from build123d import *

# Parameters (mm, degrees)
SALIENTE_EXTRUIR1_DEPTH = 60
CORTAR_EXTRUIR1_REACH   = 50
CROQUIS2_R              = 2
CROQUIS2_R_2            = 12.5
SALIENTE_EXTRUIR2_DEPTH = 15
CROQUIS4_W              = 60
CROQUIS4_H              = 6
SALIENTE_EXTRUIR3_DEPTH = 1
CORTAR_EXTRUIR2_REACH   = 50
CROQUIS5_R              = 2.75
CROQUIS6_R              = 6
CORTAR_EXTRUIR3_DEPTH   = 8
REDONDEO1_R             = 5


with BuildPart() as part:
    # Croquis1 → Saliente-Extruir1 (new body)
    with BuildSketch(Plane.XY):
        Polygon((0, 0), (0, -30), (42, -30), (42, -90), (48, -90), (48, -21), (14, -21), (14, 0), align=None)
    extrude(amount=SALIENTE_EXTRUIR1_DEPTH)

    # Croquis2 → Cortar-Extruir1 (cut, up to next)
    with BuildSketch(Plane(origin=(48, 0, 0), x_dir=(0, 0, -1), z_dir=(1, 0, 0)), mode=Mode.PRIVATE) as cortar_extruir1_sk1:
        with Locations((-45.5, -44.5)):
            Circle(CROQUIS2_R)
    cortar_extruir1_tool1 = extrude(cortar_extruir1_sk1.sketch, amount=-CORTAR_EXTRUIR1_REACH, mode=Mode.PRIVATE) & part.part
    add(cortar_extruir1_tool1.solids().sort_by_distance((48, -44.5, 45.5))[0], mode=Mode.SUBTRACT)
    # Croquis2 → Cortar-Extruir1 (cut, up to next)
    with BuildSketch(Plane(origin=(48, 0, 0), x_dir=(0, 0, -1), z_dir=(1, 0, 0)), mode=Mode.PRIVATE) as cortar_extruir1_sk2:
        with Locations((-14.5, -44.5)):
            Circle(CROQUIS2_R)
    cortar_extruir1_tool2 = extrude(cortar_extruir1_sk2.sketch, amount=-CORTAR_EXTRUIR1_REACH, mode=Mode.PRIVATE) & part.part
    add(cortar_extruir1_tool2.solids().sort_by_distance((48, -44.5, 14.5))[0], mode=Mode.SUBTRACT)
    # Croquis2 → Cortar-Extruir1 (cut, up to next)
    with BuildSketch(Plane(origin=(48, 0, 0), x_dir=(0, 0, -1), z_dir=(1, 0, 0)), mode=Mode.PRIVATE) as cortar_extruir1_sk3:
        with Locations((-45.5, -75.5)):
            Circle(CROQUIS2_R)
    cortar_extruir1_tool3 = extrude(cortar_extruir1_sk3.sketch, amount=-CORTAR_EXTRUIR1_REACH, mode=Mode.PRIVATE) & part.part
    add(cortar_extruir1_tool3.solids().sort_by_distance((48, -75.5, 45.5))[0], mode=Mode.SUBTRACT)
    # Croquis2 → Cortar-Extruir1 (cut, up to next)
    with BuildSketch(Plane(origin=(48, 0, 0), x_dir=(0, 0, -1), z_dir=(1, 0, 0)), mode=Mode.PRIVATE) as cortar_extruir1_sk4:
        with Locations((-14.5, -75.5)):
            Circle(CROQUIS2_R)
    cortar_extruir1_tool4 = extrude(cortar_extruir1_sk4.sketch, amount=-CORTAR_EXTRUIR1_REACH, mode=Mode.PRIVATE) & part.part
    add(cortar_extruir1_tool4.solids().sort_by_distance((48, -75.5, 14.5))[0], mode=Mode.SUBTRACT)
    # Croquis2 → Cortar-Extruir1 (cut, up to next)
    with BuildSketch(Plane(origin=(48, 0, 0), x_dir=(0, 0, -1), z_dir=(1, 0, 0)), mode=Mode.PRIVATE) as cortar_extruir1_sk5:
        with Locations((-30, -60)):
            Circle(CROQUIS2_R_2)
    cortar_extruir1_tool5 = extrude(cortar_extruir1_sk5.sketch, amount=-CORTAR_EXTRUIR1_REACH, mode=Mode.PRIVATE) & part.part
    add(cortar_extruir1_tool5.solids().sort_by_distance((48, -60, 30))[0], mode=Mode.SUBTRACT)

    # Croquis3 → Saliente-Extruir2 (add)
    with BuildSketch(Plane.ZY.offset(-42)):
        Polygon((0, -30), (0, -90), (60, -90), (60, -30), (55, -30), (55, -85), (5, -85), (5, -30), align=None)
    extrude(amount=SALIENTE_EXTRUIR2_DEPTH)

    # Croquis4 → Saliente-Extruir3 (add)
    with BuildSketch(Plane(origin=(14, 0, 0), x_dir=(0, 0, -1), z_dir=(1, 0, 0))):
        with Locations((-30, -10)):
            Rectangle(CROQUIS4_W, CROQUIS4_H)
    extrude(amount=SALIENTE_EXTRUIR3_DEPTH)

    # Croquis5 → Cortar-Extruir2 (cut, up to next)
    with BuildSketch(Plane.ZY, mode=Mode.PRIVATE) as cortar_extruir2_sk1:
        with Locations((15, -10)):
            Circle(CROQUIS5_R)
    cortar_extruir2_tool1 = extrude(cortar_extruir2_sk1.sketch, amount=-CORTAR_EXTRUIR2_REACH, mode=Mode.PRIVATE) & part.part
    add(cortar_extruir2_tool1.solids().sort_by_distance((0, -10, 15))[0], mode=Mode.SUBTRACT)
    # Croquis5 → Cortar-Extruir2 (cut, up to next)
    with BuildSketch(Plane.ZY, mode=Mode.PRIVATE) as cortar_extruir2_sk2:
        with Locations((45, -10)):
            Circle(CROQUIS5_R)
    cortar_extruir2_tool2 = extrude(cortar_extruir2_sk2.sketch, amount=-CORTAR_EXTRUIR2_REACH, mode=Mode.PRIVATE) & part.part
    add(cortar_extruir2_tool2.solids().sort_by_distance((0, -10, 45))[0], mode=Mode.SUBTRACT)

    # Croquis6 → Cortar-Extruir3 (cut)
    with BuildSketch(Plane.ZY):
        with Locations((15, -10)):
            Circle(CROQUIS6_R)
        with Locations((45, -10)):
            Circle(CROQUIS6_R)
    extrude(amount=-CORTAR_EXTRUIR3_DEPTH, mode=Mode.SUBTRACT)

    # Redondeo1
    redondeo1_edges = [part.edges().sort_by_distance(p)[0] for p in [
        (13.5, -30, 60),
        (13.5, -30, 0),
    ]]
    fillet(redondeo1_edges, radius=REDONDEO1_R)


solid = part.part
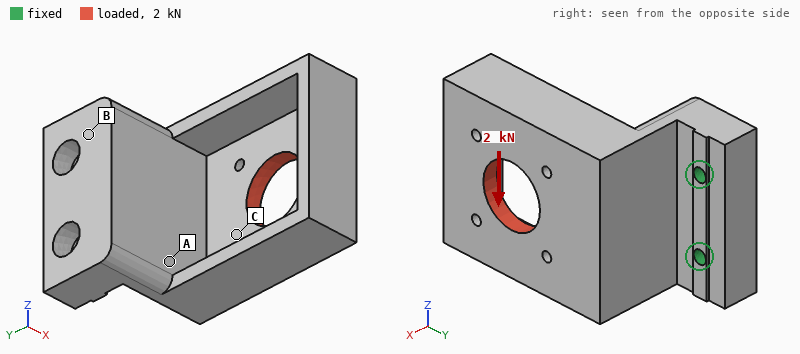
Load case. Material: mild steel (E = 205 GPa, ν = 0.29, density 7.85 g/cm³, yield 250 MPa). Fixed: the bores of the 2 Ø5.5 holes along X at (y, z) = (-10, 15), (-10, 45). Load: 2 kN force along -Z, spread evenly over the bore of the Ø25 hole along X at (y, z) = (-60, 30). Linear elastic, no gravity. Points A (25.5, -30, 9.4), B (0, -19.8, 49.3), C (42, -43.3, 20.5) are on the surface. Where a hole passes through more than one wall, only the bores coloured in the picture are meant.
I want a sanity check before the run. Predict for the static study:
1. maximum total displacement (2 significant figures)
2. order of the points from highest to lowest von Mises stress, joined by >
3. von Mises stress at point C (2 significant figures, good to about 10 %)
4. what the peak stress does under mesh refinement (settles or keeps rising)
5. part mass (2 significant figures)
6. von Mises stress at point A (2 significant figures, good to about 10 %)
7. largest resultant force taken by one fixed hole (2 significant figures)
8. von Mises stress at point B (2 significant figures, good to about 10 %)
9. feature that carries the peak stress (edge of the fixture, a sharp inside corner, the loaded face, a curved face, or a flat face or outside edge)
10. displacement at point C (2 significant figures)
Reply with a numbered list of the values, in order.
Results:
1. 100 µm
2. A > C > B
3. 30 MPa
4. keeps rising
5. 570 g
6. 45 MPa
7. 3.7 kN
8. 13 MPa
9. edge of the fixture
10. 29 µm
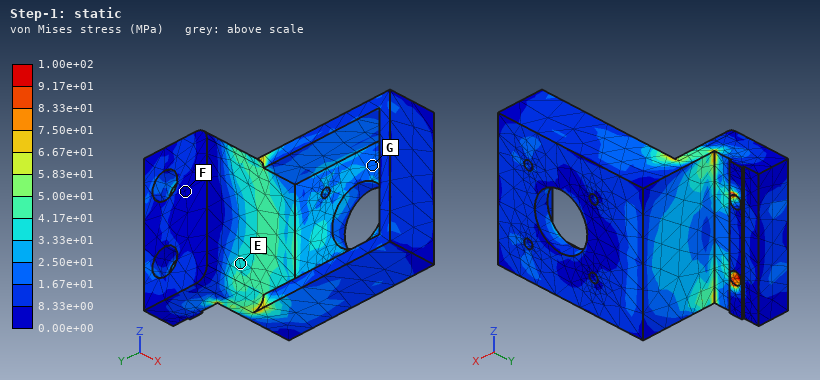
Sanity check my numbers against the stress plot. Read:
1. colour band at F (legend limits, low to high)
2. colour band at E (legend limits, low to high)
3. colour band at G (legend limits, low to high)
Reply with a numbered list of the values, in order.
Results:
1. 0.00e+00 to 8.33e+00 MPa
2. 3.33e+01 to 4.17e+01 MPa
3. 1.67e+01 to 2.50e+01 MPa
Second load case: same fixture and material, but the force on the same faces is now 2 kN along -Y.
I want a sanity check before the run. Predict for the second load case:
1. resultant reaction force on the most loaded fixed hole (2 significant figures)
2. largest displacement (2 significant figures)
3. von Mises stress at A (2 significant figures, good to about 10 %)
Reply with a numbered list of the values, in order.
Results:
1. 1.1 kN
2. 0.22 mm
3. 48 MPa
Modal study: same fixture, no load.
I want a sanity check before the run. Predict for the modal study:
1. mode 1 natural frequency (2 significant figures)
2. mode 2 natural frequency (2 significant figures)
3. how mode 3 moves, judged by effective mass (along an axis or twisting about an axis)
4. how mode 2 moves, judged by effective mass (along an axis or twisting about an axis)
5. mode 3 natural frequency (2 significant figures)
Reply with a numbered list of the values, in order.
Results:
1. 790 Hz
2. 1500 Hz
3. along Z
4. along Z
5. 3100 Hz
